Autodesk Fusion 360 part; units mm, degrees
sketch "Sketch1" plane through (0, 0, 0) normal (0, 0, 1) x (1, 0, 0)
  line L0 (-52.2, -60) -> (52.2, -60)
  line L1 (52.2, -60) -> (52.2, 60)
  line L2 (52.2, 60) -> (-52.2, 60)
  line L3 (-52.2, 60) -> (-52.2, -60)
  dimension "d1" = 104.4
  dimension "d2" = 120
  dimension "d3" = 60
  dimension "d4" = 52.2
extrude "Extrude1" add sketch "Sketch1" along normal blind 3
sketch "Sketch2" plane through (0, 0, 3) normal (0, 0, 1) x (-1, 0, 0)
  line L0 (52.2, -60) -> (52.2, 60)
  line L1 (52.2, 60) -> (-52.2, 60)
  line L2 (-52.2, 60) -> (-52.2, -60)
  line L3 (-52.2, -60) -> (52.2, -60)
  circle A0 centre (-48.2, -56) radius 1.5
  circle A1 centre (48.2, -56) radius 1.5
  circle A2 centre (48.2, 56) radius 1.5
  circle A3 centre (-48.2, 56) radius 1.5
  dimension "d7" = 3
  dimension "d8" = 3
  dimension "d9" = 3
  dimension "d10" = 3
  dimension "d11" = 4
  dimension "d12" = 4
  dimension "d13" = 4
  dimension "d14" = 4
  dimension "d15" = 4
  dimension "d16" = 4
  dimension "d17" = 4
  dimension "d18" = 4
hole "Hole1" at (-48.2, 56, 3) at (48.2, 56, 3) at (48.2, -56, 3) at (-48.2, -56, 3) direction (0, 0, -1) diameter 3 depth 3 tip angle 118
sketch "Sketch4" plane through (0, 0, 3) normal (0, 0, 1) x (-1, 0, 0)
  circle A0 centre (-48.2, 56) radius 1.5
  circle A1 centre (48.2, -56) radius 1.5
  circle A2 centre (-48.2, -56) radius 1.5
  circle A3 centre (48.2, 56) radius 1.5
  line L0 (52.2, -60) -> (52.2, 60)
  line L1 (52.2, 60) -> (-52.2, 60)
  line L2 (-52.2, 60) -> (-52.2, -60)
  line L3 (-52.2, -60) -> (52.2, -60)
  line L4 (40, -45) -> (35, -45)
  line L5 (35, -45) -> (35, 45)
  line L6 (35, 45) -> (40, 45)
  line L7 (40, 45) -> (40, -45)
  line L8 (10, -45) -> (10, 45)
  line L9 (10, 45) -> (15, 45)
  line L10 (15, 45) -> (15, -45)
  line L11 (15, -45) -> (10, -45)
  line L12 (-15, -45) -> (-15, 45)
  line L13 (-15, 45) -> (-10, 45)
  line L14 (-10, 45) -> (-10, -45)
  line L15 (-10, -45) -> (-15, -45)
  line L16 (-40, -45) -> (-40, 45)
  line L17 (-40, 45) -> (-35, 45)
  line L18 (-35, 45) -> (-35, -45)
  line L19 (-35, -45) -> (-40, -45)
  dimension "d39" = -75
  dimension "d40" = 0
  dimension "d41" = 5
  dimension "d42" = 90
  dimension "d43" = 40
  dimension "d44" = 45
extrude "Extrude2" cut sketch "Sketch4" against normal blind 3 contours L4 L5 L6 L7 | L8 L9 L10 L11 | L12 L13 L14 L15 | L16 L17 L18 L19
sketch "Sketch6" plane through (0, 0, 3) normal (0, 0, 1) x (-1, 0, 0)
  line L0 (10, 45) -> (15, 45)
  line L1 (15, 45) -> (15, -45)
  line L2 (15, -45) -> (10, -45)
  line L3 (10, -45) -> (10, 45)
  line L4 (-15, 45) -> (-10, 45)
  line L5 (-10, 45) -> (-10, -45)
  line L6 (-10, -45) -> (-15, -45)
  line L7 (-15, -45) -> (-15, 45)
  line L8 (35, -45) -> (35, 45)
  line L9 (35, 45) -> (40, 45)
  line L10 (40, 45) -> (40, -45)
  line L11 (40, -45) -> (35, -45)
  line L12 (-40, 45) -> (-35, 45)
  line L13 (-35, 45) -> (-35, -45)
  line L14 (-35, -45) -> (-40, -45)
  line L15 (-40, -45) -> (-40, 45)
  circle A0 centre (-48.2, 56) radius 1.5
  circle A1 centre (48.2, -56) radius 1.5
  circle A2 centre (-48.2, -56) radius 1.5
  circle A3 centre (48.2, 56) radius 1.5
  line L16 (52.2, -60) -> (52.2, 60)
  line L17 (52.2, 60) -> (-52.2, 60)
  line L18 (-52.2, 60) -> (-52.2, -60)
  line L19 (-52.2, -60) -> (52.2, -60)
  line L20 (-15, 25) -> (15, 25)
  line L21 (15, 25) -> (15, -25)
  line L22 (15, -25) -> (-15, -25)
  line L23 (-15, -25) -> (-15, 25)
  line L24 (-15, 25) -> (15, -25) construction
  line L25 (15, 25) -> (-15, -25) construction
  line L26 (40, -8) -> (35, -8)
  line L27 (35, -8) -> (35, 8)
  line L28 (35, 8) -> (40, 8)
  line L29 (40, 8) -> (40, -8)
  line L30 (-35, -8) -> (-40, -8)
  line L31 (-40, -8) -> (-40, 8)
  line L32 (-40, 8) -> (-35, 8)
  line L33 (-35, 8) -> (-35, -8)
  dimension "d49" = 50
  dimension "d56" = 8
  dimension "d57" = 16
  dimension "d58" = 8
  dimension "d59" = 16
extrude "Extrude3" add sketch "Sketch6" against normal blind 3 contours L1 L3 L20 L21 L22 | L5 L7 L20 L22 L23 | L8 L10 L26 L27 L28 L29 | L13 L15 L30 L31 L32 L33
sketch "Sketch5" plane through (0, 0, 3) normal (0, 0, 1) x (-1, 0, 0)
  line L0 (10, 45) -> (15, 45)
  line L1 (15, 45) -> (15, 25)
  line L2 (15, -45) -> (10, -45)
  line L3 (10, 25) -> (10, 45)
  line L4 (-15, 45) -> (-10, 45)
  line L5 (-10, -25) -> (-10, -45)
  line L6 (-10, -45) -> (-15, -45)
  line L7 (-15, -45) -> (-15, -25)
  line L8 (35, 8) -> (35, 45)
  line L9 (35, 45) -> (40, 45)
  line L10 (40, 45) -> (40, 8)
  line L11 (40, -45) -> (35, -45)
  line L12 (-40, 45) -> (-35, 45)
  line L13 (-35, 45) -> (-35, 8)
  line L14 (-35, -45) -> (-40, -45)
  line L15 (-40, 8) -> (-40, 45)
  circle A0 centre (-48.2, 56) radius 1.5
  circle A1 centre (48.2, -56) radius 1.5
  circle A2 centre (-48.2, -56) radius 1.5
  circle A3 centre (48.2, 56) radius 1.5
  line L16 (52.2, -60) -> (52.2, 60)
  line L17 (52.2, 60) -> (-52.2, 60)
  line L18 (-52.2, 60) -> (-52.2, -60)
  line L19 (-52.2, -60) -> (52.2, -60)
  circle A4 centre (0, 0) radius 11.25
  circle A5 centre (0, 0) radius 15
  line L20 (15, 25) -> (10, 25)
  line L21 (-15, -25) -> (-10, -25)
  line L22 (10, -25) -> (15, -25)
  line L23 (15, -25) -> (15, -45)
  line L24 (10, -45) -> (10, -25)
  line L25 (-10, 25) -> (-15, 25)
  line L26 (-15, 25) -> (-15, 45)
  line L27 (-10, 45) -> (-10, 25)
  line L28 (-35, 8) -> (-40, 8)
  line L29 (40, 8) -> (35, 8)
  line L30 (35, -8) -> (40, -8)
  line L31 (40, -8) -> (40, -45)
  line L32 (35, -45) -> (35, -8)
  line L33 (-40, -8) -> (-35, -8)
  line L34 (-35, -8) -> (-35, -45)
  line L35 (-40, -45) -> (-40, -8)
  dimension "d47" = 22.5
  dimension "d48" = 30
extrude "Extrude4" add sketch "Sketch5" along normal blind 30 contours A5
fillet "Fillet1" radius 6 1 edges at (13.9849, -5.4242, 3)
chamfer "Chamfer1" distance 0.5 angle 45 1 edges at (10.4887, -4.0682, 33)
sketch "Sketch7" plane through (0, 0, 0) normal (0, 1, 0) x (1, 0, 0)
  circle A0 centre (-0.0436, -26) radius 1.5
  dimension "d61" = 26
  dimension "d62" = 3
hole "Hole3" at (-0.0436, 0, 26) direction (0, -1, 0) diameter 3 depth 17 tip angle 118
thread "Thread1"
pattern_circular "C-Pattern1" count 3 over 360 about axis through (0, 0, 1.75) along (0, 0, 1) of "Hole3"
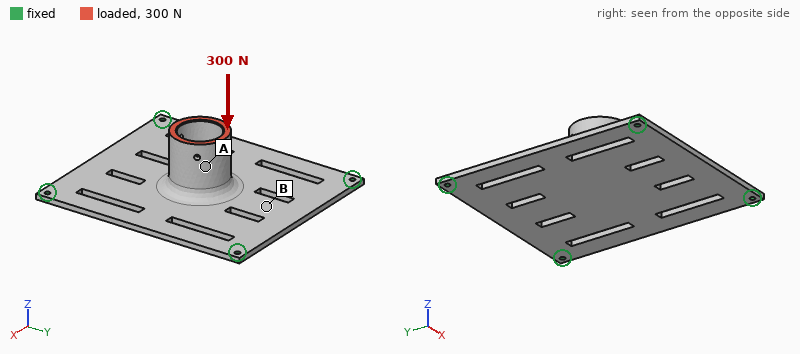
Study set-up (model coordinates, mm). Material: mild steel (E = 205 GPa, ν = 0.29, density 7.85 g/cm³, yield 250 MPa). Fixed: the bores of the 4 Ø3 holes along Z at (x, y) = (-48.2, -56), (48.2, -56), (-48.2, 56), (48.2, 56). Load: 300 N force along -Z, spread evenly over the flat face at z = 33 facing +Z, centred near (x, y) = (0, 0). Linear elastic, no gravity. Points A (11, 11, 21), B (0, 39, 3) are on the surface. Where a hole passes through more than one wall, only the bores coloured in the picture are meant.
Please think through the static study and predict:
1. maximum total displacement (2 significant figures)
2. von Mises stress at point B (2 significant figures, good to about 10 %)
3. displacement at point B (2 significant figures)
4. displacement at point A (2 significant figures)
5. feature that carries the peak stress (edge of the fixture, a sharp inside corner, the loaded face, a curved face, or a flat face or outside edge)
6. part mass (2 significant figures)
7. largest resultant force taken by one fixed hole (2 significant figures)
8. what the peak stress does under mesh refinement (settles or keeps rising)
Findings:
84 µm
9.4 MPa
61 µm
83 µm
edge of the fixture
350 g
77 N
keeps rising
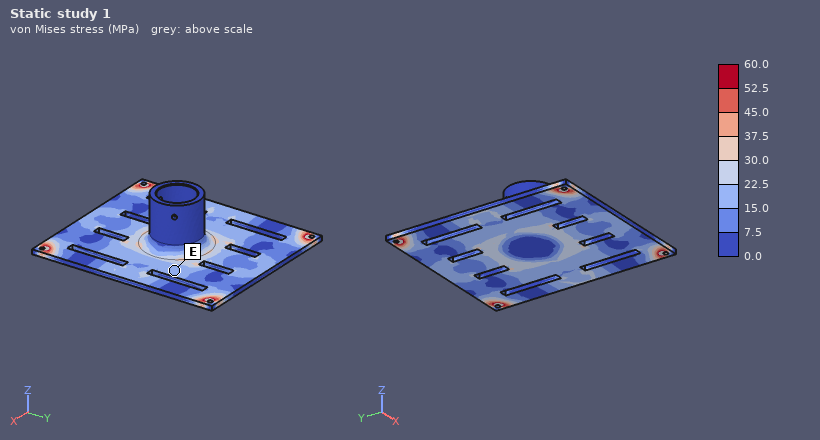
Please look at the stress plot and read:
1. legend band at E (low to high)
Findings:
15.0 to 22.5 MPa
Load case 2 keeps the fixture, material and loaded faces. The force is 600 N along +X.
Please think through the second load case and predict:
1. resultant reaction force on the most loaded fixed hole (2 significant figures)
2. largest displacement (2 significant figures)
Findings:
210 N
0.13 mm
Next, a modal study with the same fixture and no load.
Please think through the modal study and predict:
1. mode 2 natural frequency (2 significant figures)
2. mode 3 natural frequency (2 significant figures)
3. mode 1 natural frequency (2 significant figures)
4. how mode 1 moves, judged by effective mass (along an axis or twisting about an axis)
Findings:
1200 Hz
1300 Hz
670 Hz
along Z
